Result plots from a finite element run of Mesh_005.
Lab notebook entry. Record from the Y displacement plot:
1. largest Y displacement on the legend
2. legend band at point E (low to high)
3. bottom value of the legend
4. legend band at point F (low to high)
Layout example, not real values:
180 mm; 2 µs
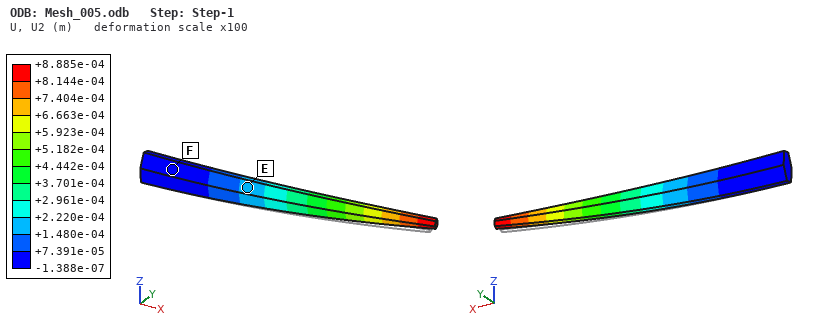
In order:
+8.885e-04 m; +1.480e-04 to +2.220e-04 m; -1.388e-07 m; -1.388e-07 to +7.391e-05 m
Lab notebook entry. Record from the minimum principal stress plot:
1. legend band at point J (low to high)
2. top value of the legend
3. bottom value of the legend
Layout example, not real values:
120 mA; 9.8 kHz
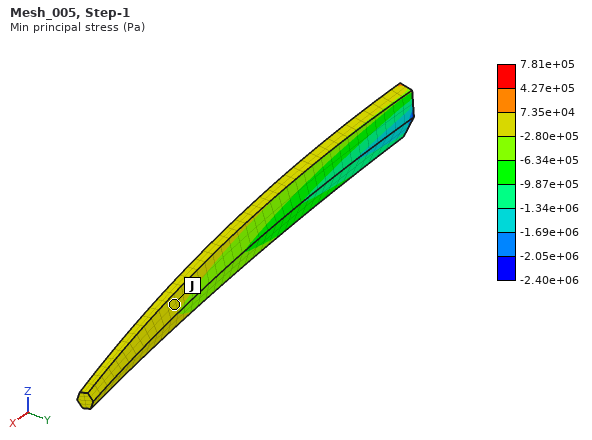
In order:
-2.80e+05 to 7.35e+04 Pa; 7.81e+05 Pa; -2.40e+06 Pa
